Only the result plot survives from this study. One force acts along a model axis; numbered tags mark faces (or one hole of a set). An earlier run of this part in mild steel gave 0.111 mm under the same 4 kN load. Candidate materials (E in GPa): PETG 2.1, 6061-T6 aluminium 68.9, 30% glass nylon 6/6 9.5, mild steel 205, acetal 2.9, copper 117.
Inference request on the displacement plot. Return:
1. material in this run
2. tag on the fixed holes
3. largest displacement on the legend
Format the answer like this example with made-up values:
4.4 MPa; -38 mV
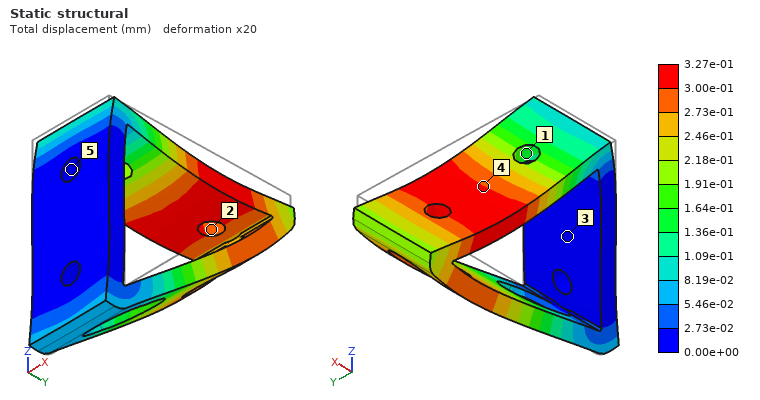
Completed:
6061-T6 aluminium; 5; 3.27e-01 mm
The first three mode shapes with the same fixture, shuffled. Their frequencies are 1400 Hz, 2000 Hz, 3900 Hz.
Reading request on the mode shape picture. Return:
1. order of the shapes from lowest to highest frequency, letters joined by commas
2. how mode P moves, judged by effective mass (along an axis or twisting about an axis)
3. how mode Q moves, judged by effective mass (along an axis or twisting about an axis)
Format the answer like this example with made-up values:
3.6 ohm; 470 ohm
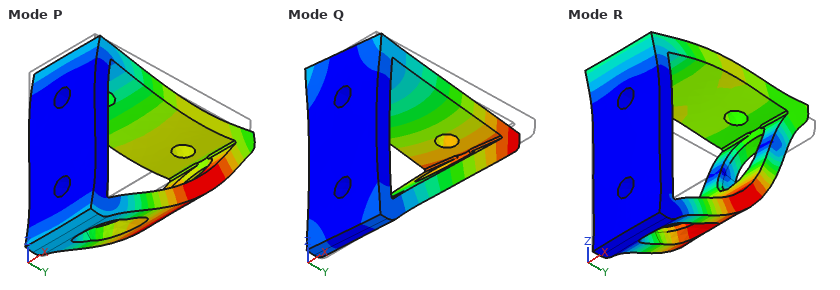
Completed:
Q, P, R; along Z; along X
